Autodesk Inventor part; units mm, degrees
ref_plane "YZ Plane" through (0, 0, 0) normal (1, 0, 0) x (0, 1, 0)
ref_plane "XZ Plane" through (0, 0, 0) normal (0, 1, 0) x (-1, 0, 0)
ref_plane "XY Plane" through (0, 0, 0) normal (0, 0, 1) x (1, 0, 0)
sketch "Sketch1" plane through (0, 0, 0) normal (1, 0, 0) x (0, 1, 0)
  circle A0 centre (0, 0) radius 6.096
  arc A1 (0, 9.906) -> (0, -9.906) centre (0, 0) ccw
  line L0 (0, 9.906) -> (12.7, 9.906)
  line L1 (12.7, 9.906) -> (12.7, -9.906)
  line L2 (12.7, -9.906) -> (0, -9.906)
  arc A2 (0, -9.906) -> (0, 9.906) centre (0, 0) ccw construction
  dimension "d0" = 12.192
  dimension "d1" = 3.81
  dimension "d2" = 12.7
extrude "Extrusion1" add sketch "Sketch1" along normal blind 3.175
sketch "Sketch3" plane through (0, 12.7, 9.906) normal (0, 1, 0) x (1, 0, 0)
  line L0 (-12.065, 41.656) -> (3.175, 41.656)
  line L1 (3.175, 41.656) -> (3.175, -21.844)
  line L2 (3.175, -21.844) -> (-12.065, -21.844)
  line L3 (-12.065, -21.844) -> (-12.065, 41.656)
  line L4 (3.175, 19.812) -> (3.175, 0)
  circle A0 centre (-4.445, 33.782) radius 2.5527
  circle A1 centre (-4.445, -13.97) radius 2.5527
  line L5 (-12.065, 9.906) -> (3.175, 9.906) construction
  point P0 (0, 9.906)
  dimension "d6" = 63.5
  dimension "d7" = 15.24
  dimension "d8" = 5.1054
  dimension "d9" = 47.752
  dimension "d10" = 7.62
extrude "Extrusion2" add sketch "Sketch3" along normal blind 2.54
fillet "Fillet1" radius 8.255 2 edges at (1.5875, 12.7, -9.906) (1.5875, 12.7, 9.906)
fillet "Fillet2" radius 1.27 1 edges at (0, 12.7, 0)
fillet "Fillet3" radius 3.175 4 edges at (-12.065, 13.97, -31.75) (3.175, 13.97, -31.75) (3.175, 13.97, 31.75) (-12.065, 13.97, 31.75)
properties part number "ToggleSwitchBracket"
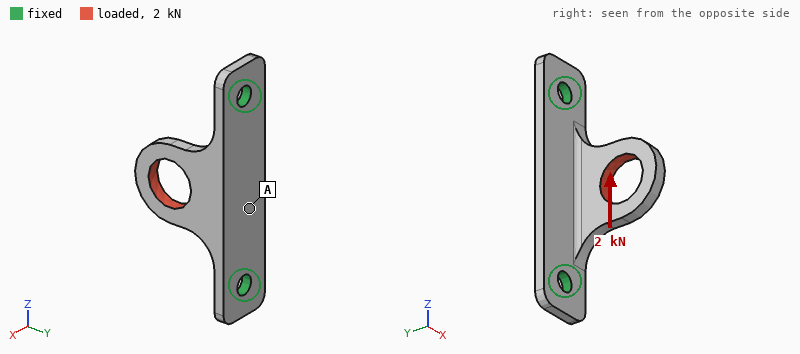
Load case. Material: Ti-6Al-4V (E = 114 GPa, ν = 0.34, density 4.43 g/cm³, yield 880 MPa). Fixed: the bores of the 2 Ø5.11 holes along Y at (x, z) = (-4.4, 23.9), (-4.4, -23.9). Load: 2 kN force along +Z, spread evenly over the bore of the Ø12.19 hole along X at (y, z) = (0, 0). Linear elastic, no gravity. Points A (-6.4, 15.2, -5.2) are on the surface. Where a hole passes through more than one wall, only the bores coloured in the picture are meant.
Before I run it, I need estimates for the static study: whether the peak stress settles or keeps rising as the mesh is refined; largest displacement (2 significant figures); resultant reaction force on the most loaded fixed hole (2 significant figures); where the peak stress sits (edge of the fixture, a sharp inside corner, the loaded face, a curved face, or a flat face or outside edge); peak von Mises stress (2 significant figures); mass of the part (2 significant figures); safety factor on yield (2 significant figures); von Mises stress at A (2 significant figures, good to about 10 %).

settles
0.16 mm
1.3 kN
a curved face
550 MPa
15 g
1.6
48 MPa
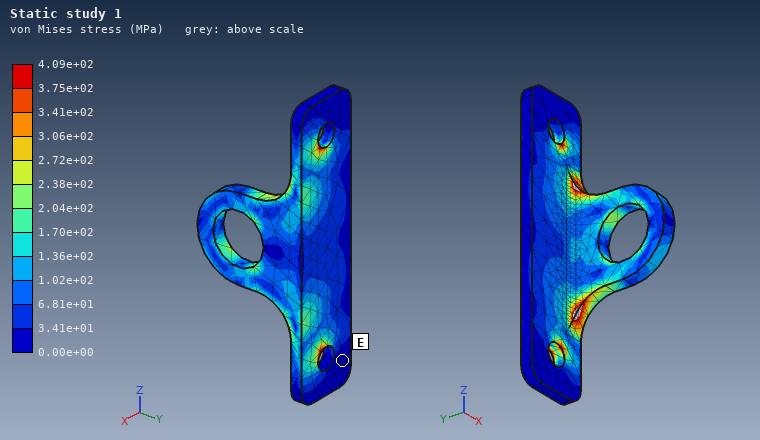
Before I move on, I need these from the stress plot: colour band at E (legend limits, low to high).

0.00e+00 to 3.41e+01 MPa
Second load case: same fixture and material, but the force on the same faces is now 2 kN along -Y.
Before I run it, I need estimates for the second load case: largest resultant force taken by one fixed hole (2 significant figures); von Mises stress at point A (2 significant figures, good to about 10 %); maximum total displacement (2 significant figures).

1.3 kN
48 MPa
0.34 mm
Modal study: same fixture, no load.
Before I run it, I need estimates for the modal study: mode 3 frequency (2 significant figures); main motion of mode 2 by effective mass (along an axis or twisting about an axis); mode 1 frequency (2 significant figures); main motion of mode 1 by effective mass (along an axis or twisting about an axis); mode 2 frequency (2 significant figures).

11 kHz
along Y
3600 Hz
along X
7500 Hz
